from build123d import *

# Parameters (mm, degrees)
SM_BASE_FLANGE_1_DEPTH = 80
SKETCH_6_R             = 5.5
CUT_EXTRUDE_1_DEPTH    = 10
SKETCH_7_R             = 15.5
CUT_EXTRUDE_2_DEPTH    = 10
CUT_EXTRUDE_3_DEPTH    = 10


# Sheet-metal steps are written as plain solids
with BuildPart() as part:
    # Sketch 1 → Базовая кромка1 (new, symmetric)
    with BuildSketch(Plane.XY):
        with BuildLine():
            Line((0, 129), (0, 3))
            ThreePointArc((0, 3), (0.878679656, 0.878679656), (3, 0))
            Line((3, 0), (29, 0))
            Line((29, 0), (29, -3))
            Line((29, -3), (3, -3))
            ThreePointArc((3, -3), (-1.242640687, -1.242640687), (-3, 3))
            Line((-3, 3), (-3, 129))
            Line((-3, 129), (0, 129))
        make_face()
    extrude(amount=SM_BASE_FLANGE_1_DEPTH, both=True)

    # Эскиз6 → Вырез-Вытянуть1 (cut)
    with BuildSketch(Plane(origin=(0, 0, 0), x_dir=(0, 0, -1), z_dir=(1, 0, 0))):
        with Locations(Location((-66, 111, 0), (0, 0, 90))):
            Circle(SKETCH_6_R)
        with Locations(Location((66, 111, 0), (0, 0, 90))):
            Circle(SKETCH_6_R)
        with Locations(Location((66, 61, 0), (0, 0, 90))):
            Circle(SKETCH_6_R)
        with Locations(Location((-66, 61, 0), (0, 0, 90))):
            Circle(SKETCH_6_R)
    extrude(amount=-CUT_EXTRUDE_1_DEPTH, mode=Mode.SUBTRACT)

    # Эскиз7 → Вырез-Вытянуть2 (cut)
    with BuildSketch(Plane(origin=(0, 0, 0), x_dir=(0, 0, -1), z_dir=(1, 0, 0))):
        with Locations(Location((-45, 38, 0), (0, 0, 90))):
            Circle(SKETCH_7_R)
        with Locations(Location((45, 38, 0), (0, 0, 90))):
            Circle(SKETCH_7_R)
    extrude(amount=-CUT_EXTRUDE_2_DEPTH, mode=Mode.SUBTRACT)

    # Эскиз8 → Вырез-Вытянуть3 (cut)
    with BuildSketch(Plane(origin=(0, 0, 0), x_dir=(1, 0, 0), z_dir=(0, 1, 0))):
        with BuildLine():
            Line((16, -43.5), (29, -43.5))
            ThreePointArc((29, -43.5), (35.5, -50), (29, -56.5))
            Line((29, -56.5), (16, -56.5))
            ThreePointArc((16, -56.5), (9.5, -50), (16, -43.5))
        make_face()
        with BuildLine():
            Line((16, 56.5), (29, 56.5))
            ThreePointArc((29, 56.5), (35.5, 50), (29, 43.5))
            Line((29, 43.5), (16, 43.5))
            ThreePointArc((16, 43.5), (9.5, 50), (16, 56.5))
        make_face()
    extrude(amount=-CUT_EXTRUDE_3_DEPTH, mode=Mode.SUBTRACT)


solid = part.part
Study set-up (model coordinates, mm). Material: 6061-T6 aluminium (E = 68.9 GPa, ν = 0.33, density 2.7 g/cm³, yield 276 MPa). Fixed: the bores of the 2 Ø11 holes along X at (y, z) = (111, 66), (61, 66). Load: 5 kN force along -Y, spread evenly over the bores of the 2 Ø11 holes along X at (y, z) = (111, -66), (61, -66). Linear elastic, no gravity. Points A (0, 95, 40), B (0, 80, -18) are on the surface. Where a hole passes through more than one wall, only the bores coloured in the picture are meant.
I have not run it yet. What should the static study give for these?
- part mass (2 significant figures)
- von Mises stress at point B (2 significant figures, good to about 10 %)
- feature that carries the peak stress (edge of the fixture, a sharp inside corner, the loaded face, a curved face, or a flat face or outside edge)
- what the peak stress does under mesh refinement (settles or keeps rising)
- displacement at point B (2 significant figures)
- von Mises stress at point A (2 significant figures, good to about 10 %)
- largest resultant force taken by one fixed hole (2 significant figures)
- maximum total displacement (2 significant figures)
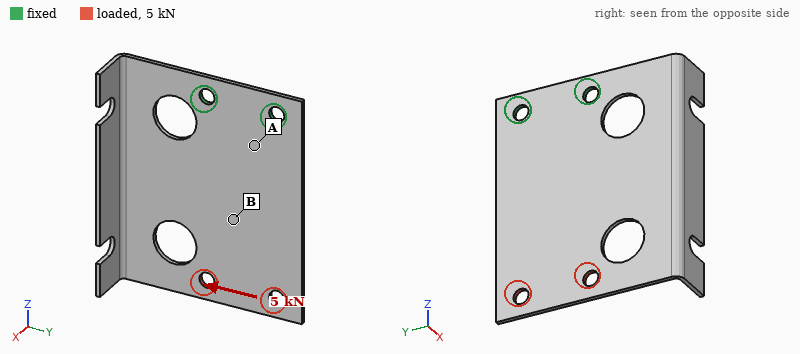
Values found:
190 g
36 MPa
edge of the fixture
keeps rising
0.27 mm
81 MPa
12 kN
0.61 mm
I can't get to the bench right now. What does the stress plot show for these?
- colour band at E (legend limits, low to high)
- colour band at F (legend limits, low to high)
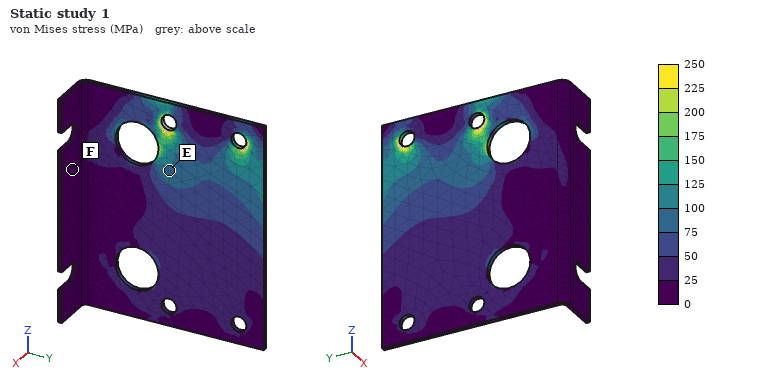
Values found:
75 to 100 MPa
0 to 25 MPa
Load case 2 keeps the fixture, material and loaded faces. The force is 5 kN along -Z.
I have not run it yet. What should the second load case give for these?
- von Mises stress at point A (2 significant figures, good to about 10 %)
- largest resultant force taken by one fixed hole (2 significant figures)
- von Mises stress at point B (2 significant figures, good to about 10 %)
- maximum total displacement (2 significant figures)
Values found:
17 MPa
2.5 kN
20 MPa
51 µm
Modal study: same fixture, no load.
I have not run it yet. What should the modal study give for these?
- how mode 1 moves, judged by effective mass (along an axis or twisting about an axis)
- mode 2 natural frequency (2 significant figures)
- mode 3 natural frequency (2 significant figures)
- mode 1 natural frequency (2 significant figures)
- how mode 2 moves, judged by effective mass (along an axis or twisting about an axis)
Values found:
along X
210 Hz
440 Hz
100 Hz
twisting about Z
